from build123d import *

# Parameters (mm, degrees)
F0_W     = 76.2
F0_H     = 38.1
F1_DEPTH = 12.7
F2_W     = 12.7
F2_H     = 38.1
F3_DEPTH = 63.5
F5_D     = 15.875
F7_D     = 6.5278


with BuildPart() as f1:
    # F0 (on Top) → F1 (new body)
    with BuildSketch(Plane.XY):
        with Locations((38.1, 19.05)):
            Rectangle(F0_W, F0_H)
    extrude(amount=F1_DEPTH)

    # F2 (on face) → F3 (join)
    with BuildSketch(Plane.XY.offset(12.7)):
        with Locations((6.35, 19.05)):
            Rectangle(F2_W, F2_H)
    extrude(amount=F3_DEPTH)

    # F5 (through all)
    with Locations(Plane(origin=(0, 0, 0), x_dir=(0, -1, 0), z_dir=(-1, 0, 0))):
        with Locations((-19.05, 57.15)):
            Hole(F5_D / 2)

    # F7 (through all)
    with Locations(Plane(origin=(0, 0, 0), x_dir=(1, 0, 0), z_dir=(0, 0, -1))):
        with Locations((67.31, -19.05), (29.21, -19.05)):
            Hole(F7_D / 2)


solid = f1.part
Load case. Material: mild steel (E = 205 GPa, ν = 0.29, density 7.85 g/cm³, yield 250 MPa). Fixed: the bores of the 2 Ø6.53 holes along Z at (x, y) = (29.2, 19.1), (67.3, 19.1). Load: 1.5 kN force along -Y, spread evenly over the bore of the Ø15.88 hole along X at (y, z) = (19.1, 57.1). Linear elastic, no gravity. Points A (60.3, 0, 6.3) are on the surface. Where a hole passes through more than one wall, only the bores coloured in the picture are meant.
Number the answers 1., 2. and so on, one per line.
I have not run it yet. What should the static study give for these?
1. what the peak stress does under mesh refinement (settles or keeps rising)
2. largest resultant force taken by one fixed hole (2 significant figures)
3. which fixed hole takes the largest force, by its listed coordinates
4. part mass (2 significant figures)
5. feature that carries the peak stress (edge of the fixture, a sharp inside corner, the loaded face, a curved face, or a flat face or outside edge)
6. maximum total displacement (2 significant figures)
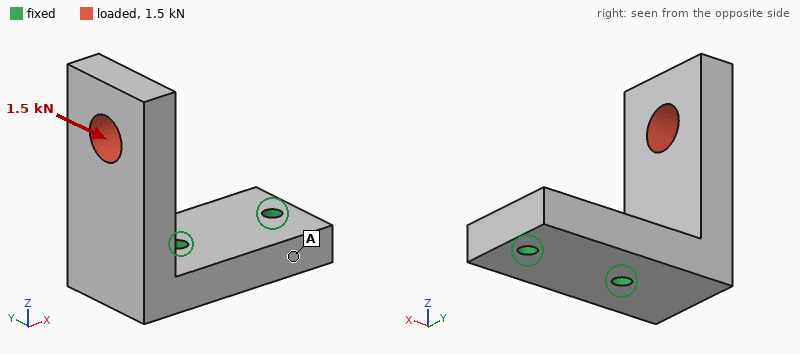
1. keeps rising
2. 2.2 kN
3. (29.2, 19.1)
4. 500 g
5. edge of the fixture
6. 79 µm
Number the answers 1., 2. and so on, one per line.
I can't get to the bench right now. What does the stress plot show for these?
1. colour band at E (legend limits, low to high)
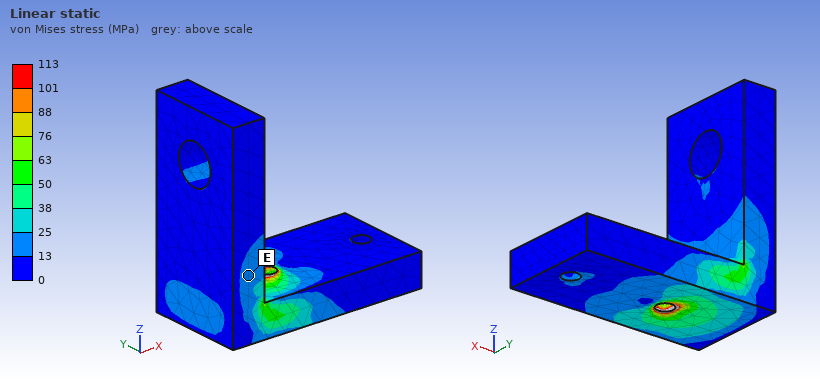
1. 13 to 25 MPa
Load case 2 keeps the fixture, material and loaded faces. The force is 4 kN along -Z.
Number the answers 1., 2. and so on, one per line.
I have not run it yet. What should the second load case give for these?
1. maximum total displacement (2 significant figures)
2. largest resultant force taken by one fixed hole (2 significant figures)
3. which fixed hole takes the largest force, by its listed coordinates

1. 71 µm
2. 4.7 kN
3. (29.2, 19.1)
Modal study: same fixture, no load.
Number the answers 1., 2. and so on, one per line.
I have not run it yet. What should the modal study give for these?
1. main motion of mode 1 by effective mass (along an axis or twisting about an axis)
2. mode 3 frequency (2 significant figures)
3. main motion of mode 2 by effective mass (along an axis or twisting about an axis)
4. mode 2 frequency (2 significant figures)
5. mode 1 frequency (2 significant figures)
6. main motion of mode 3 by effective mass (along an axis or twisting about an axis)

1. along X
2. 5700 Hz
3. along Y
4. 2100 Hz
5. 1500 Hz
6. along Z
